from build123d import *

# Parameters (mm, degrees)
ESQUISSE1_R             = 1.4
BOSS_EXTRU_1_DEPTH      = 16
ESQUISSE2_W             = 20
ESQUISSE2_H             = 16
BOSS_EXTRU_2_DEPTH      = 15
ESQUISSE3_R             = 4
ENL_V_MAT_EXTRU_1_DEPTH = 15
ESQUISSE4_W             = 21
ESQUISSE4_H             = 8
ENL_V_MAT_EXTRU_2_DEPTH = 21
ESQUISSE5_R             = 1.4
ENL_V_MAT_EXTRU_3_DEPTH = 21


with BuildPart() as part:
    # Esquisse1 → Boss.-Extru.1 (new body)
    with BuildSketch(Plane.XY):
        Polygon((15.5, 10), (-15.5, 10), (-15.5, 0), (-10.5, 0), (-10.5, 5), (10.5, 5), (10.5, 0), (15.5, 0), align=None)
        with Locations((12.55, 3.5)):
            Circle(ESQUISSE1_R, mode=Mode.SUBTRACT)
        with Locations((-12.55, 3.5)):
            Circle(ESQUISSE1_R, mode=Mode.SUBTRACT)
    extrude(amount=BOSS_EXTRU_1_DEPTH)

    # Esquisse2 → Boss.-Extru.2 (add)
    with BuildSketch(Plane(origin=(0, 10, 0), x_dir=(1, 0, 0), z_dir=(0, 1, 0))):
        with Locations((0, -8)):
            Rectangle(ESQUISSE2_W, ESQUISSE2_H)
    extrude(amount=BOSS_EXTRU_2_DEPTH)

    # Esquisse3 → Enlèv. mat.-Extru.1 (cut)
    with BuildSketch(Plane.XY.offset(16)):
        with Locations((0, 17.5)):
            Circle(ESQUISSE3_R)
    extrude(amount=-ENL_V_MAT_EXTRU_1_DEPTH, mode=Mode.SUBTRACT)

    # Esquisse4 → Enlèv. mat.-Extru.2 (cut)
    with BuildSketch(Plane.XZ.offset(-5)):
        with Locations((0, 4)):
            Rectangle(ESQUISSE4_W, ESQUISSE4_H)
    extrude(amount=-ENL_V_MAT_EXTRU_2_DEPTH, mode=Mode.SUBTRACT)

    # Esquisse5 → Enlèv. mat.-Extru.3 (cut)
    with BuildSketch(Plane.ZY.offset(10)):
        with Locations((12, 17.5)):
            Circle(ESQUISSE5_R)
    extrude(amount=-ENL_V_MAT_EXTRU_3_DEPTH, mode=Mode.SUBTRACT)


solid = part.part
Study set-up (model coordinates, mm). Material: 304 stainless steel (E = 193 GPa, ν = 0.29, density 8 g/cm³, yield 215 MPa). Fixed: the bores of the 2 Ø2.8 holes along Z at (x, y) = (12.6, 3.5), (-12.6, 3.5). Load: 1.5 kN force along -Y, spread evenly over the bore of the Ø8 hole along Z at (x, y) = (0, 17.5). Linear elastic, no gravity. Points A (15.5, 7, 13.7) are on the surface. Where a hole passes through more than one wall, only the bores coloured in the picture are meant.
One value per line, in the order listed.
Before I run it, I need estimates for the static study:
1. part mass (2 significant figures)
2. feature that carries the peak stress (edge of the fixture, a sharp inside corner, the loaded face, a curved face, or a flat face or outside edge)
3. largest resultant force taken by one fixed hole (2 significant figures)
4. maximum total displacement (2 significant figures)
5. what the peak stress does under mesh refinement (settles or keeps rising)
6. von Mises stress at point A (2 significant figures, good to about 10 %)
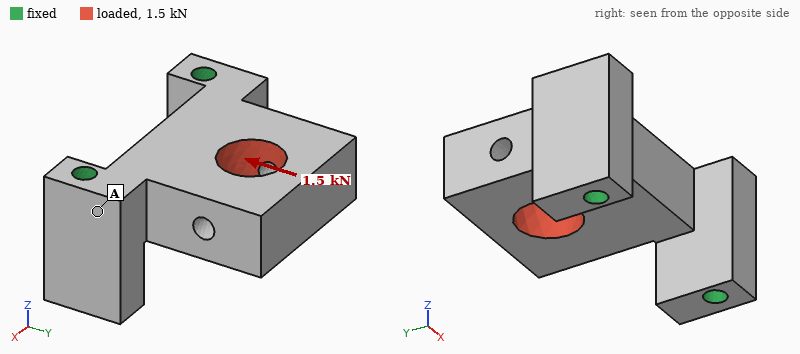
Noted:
33 g
edge of the fixture
880 N
3.0 µm
keeps rising
7.4 MPa
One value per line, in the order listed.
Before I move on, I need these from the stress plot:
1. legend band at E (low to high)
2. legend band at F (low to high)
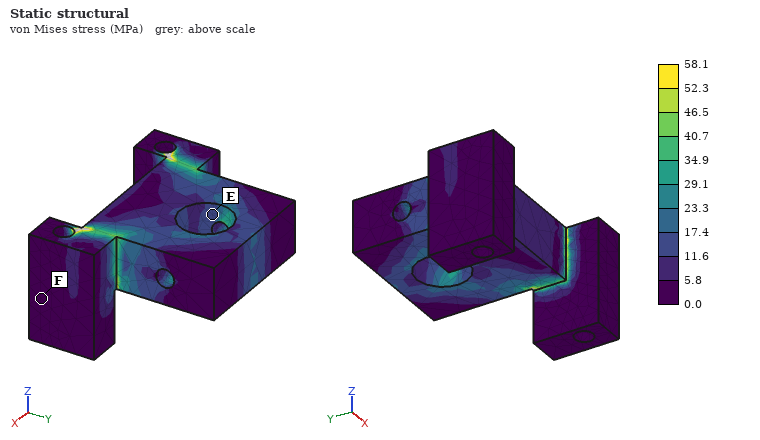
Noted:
11.6 to 17.4 MPa
0.0 to 5.8 MPa
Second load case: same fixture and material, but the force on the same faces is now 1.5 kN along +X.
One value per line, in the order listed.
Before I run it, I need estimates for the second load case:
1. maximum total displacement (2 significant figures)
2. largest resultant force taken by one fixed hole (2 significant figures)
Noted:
6.1 µm
1.1 kN
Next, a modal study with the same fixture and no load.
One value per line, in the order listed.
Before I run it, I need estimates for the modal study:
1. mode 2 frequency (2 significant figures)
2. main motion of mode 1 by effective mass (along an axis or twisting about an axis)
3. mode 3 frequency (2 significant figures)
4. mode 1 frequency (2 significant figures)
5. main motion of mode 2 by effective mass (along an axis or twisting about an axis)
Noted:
23 kHz
along Z
24 kHz
9400 Hz
along X
